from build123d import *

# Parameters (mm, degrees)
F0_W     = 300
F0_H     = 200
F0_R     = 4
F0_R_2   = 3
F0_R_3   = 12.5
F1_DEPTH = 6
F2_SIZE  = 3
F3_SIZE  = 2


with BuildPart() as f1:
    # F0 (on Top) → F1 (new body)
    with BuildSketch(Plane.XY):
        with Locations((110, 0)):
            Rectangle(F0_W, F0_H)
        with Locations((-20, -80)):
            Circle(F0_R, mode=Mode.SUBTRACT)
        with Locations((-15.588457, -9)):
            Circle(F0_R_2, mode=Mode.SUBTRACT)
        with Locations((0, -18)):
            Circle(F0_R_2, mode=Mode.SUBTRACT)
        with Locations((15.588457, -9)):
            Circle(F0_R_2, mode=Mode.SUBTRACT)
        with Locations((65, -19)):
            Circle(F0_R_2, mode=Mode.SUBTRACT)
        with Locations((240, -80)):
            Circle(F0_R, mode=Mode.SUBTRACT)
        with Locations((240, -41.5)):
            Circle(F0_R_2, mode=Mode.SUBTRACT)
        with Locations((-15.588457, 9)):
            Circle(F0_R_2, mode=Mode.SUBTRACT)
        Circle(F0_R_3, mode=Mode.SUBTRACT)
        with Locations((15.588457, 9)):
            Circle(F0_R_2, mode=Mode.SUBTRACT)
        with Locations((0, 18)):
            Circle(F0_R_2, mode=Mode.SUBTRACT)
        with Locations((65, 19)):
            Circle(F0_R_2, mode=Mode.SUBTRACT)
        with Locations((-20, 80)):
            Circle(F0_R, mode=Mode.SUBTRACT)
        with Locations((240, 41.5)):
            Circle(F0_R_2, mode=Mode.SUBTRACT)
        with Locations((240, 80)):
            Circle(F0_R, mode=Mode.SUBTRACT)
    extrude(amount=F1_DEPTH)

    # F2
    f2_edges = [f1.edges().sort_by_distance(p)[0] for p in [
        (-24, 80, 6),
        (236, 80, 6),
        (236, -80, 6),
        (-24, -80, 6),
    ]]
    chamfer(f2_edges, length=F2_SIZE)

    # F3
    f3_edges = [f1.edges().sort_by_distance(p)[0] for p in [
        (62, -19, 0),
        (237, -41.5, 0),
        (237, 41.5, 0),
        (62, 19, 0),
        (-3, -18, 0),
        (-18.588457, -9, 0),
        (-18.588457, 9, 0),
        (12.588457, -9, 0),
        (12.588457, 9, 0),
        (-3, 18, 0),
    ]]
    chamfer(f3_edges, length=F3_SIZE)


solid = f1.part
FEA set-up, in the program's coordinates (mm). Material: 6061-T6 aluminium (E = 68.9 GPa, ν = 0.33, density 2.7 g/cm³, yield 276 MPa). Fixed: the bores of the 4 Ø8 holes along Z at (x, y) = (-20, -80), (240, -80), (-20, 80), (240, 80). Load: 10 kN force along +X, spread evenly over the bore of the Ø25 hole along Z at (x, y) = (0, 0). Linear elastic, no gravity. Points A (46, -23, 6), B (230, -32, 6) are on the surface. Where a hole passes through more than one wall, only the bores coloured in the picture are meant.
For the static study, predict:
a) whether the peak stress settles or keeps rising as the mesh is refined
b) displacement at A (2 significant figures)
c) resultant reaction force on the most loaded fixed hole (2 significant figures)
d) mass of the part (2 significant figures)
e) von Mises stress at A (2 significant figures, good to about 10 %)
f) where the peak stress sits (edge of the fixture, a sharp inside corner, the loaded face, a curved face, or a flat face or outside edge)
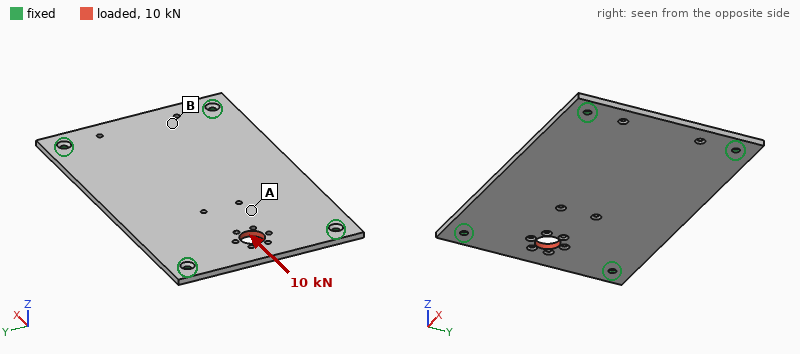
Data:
keeps rising
23 µm
3.3 kN
950 g
14 MPa
edge of the fixture
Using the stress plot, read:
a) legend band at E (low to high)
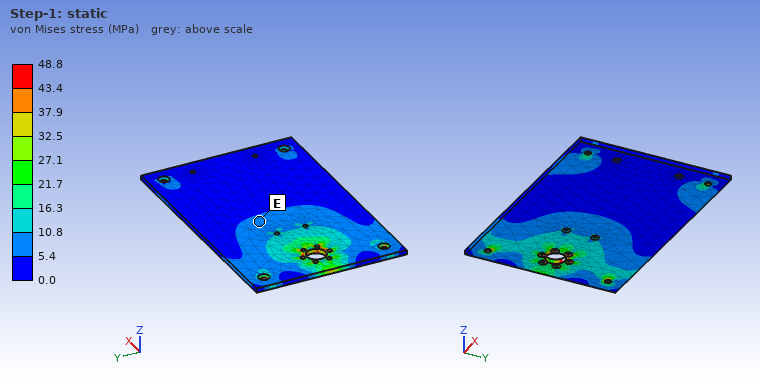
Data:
5.4 to 10.8 MPa
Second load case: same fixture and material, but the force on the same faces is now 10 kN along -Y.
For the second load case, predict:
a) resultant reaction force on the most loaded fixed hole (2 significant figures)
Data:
4.5 kN
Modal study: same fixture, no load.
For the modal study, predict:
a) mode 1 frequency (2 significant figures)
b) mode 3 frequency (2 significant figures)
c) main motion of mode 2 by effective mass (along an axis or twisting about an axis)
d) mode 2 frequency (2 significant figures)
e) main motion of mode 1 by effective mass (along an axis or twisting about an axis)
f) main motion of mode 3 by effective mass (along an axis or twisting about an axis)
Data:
350 Hz
900 Hz
twisting about X
560 Hz
along Z
twisting about Y
